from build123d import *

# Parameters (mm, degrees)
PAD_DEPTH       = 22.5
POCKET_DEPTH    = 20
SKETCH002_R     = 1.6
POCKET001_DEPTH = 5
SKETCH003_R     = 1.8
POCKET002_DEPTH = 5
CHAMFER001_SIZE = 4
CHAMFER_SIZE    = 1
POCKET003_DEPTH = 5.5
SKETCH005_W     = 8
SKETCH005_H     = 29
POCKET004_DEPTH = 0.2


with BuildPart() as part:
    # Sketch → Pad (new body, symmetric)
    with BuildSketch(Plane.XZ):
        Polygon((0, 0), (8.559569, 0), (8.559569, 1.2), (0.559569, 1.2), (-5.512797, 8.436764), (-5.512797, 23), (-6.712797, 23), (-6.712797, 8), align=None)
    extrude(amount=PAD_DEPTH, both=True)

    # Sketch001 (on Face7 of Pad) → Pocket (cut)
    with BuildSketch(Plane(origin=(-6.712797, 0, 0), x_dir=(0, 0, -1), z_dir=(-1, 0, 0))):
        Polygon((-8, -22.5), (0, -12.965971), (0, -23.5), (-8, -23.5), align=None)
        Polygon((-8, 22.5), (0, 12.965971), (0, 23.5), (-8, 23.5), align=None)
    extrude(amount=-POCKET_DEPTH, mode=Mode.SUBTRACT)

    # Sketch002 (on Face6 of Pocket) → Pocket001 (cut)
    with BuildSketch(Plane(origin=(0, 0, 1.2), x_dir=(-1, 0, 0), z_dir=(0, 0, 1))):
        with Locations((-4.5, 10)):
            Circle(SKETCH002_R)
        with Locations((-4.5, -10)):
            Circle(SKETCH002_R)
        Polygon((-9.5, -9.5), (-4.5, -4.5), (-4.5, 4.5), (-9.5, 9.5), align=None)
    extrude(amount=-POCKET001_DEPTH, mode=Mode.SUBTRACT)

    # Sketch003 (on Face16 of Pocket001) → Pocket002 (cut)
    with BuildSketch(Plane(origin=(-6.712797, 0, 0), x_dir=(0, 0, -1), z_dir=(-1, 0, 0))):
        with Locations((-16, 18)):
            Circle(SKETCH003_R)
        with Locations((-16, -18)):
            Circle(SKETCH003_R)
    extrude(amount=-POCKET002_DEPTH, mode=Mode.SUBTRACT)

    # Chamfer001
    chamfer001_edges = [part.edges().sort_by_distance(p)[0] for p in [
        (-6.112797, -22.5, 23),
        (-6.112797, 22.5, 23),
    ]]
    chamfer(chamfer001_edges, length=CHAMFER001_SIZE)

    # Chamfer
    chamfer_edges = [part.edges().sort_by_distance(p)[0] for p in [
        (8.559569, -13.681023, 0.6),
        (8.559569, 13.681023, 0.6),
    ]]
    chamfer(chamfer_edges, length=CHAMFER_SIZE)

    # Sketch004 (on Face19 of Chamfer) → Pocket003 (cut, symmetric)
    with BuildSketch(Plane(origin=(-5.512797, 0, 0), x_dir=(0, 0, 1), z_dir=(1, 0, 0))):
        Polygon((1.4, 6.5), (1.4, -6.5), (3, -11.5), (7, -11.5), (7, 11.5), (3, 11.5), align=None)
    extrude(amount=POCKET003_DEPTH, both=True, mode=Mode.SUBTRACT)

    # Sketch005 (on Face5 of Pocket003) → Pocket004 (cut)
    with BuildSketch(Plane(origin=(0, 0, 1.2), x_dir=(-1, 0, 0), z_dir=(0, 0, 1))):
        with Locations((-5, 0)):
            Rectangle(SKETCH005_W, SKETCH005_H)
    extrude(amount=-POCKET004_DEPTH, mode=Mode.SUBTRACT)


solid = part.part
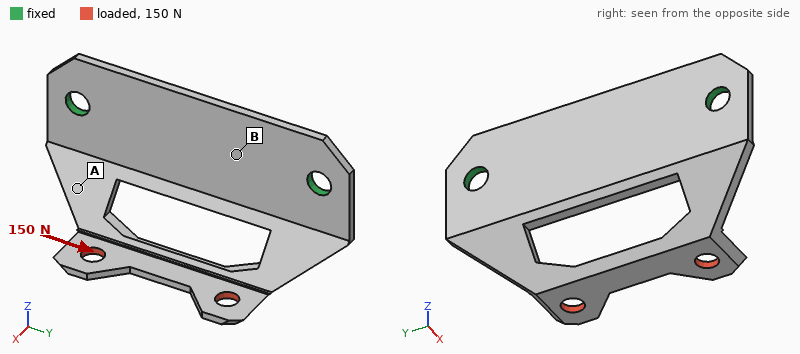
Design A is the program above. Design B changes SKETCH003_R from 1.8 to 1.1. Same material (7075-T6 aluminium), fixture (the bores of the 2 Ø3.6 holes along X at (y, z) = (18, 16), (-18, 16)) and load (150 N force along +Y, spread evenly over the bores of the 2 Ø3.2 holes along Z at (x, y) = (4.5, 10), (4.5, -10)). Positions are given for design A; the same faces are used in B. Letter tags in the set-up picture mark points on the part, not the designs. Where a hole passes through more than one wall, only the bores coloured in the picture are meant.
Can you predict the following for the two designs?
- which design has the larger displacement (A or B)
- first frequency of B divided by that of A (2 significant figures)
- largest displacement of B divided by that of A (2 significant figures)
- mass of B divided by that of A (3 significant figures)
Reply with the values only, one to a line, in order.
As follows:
B
0.94
1.1
1.01
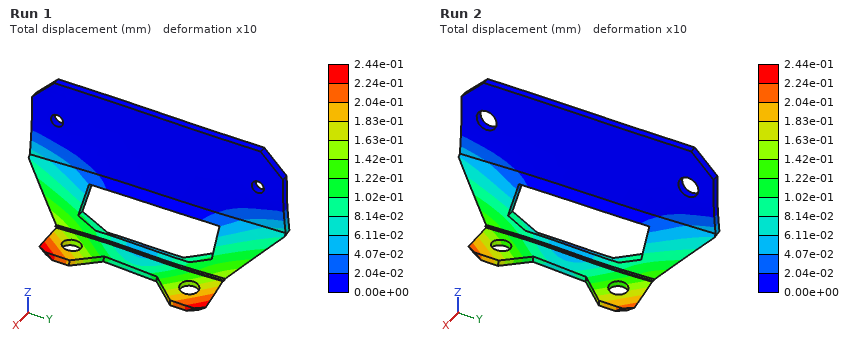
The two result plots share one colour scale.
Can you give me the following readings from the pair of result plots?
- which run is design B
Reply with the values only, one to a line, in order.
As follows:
Run 1
